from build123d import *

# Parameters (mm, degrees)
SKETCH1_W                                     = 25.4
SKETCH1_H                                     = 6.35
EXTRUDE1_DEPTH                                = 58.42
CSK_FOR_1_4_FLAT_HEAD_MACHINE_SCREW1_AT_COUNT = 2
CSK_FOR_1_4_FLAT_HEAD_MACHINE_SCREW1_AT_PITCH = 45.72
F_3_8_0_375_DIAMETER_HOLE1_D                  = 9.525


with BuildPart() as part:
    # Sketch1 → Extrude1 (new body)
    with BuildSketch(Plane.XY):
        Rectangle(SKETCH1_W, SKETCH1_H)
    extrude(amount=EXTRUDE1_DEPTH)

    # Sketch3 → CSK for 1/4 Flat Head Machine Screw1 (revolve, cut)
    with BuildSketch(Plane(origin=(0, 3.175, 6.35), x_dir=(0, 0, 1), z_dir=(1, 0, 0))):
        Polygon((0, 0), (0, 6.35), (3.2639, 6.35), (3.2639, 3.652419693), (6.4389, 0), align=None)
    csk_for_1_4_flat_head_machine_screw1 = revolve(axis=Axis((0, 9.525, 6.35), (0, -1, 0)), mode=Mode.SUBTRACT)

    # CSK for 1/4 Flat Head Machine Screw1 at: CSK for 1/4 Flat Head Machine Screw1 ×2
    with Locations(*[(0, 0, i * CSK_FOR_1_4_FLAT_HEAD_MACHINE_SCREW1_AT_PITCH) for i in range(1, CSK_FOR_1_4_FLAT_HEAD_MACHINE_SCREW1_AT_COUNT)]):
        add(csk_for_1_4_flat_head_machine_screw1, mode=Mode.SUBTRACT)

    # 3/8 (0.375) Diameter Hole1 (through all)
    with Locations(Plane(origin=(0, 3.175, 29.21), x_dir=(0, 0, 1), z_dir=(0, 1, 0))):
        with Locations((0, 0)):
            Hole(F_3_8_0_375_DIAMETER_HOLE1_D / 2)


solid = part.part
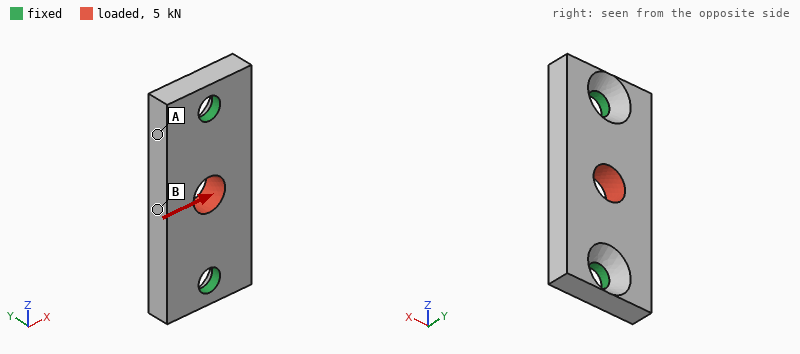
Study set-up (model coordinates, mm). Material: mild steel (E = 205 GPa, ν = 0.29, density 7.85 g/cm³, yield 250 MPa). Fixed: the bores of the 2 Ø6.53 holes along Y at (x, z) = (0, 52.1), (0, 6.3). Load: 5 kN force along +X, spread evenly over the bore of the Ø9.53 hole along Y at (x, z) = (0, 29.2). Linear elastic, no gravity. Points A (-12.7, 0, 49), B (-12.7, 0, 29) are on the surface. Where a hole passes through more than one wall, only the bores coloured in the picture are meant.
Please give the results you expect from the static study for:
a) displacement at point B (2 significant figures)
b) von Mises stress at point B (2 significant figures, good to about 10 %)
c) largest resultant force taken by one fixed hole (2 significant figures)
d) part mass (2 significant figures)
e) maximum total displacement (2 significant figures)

11 µm
72 MPa
2.5 kN
65 g
12 µm
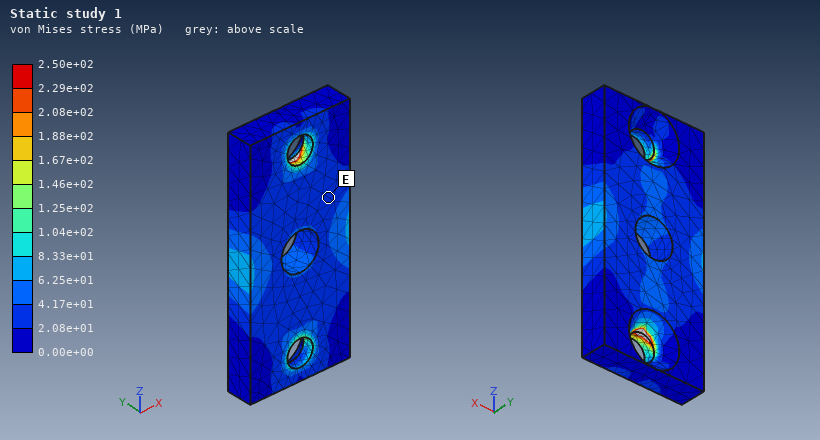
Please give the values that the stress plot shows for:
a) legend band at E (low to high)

2.08e+01 to 4.17e+01 MPa
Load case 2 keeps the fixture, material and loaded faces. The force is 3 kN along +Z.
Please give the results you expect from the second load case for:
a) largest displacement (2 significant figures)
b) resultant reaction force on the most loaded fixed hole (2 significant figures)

2.0 µm
1.5 kN
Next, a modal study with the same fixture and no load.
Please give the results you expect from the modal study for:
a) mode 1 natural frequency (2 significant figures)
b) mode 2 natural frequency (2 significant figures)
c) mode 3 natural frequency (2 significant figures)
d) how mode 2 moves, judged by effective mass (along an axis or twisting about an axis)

11 kHz
11 kHz
20 kHz
along Y
